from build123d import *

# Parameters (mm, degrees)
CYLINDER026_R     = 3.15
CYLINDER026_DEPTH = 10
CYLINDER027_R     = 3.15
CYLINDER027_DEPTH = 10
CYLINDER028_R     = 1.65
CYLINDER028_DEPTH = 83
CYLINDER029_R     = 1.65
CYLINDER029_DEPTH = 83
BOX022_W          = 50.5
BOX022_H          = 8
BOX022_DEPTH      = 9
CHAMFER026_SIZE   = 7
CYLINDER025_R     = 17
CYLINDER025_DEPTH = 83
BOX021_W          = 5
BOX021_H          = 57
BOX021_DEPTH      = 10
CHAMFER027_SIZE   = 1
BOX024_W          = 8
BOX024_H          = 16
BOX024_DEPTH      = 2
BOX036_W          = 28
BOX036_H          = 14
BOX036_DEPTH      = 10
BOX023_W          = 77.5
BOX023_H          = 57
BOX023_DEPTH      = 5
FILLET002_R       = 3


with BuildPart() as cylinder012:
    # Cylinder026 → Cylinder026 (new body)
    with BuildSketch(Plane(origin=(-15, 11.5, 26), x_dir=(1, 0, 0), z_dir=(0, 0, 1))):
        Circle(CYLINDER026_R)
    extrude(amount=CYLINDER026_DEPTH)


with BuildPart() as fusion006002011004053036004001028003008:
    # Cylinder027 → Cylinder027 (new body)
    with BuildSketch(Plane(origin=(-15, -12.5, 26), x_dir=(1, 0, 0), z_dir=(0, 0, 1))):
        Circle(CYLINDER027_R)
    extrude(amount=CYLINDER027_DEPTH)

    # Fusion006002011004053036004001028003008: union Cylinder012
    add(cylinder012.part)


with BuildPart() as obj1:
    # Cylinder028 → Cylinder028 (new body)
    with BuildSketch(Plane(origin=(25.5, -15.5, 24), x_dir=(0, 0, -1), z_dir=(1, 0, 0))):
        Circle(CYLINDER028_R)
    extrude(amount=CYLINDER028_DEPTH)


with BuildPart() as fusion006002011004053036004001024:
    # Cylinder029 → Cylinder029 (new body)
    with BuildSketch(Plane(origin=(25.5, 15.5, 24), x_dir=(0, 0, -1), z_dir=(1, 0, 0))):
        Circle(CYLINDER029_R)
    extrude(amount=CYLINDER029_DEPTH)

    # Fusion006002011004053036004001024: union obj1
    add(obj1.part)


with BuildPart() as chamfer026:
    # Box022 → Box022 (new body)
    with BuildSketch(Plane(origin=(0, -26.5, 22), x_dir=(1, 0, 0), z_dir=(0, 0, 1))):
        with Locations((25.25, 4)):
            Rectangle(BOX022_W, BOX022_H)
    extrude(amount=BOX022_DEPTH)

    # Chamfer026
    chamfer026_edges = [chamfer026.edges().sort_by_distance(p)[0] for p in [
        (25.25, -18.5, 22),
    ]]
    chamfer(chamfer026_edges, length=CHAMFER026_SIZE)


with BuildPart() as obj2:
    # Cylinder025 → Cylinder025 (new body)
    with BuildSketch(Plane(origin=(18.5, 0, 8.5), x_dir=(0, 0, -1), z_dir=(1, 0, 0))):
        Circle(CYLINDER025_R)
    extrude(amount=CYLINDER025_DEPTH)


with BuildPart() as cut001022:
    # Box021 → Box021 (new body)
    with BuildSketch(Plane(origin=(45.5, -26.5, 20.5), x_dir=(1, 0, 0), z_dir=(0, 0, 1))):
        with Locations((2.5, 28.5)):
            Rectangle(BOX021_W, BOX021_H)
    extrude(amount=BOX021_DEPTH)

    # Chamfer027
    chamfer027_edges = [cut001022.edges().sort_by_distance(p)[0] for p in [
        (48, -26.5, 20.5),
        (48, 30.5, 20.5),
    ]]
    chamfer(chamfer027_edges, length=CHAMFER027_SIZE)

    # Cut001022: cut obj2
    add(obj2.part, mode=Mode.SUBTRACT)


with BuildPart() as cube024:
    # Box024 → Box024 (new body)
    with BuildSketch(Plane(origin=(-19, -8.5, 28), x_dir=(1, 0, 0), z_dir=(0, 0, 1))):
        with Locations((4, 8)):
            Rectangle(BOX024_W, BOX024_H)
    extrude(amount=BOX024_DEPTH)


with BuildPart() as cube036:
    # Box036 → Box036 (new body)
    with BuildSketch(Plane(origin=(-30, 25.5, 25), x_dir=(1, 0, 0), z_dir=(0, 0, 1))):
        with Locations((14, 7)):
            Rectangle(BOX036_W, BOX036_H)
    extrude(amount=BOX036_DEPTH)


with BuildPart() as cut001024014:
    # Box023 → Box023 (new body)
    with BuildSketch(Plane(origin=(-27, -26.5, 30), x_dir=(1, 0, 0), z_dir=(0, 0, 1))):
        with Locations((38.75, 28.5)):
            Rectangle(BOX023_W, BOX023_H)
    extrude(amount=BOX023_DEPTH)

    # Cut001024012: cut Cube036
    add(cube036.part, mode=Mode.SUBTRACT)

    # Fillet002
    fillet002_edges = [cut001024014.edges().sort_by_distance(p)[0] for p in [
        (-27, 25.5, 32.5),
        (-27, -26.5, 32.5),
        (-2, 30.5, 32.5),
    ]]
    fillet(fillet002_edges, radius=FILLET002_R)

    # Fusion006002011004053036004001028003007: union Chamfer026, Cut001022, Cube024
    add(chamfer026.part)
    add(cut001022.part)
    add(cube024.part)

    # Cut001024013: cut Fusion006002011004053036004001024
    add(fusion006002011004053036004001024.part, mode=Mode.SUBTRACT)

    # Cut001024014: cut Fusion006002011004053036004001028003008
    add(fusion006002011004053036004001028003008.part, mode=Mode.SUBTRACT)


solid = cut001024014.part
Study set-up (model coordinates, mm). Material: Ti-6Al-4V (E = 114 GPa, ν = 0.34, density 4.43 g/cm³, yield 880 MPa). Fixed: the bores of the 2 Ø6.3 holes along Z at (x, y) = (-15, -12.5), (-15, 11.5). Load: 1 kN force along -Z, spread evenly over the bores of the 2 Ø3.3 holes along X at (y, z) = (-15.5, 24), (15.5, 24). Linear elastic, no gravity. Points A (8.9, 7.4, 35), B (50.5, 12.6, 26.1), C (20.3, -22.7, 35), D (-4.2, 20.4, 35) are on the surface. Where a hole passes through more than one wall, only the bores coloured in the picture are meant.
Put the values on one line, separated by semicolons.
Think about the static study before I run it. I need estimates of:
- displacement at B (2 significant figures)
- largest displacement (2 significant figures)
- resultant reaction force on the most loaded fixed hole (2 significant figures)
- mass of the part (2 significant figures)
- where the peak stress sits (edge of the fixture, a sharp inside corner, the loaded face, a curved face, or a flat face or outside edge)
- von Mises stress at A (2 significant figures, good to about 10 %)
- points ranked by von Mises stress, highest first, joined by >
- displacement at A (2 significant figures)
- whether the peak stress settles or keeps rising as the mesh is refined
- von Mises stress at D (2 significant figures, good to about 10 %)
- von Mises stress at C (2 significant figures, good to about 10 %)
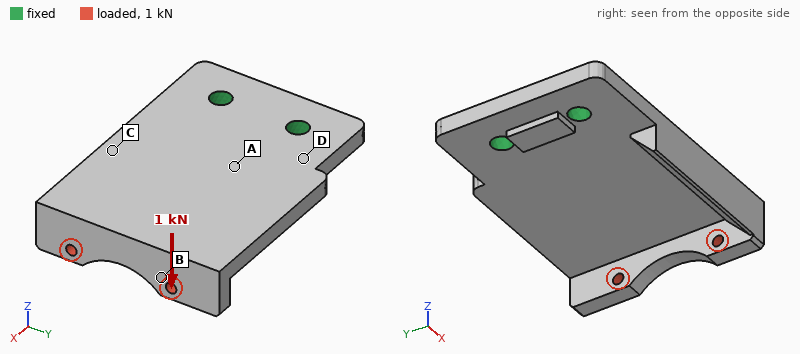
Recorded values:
1.1 mm; 1.1 mm; 640 N; 110 g; edge of the fixture; 120 MPa; D > A > C > B; 0.21 mm; keeps rising; 200 MPa; 65 MPa
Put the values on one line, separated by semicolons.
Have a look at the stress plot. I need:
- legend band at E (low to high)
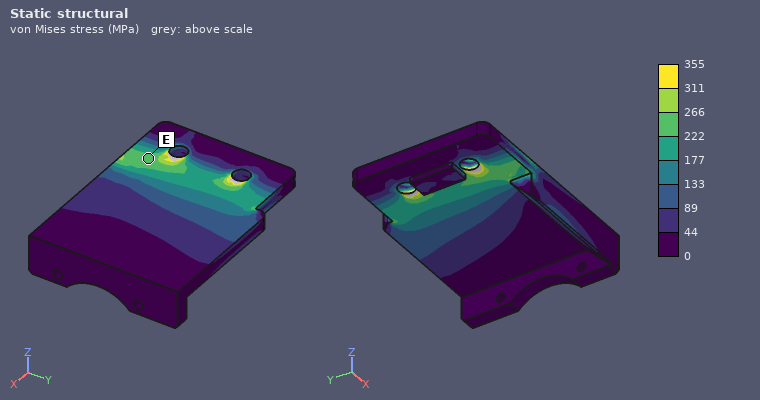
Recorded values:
222 to 266 MPa
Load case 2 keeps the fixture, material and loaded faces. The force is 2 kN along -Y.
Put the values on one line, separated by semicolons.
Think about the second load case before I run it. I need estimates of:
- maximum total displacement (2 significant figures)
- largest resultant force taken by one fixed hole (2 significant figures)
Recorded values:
0.24 mm; 4.5 kN
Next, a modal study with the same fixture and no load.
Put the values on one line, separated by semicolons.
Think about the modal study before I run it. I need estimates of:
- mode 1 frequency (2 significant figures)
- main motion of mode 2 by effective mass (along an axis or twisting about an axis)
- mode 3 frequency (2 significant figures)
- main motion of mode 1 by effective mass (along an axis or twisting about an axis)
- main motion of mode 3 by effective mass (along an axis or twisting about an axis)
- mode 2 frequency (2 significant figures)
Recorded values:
840 Hz; twisting about X; 4800 Hz; along Z; along Y; 2000 Hz
